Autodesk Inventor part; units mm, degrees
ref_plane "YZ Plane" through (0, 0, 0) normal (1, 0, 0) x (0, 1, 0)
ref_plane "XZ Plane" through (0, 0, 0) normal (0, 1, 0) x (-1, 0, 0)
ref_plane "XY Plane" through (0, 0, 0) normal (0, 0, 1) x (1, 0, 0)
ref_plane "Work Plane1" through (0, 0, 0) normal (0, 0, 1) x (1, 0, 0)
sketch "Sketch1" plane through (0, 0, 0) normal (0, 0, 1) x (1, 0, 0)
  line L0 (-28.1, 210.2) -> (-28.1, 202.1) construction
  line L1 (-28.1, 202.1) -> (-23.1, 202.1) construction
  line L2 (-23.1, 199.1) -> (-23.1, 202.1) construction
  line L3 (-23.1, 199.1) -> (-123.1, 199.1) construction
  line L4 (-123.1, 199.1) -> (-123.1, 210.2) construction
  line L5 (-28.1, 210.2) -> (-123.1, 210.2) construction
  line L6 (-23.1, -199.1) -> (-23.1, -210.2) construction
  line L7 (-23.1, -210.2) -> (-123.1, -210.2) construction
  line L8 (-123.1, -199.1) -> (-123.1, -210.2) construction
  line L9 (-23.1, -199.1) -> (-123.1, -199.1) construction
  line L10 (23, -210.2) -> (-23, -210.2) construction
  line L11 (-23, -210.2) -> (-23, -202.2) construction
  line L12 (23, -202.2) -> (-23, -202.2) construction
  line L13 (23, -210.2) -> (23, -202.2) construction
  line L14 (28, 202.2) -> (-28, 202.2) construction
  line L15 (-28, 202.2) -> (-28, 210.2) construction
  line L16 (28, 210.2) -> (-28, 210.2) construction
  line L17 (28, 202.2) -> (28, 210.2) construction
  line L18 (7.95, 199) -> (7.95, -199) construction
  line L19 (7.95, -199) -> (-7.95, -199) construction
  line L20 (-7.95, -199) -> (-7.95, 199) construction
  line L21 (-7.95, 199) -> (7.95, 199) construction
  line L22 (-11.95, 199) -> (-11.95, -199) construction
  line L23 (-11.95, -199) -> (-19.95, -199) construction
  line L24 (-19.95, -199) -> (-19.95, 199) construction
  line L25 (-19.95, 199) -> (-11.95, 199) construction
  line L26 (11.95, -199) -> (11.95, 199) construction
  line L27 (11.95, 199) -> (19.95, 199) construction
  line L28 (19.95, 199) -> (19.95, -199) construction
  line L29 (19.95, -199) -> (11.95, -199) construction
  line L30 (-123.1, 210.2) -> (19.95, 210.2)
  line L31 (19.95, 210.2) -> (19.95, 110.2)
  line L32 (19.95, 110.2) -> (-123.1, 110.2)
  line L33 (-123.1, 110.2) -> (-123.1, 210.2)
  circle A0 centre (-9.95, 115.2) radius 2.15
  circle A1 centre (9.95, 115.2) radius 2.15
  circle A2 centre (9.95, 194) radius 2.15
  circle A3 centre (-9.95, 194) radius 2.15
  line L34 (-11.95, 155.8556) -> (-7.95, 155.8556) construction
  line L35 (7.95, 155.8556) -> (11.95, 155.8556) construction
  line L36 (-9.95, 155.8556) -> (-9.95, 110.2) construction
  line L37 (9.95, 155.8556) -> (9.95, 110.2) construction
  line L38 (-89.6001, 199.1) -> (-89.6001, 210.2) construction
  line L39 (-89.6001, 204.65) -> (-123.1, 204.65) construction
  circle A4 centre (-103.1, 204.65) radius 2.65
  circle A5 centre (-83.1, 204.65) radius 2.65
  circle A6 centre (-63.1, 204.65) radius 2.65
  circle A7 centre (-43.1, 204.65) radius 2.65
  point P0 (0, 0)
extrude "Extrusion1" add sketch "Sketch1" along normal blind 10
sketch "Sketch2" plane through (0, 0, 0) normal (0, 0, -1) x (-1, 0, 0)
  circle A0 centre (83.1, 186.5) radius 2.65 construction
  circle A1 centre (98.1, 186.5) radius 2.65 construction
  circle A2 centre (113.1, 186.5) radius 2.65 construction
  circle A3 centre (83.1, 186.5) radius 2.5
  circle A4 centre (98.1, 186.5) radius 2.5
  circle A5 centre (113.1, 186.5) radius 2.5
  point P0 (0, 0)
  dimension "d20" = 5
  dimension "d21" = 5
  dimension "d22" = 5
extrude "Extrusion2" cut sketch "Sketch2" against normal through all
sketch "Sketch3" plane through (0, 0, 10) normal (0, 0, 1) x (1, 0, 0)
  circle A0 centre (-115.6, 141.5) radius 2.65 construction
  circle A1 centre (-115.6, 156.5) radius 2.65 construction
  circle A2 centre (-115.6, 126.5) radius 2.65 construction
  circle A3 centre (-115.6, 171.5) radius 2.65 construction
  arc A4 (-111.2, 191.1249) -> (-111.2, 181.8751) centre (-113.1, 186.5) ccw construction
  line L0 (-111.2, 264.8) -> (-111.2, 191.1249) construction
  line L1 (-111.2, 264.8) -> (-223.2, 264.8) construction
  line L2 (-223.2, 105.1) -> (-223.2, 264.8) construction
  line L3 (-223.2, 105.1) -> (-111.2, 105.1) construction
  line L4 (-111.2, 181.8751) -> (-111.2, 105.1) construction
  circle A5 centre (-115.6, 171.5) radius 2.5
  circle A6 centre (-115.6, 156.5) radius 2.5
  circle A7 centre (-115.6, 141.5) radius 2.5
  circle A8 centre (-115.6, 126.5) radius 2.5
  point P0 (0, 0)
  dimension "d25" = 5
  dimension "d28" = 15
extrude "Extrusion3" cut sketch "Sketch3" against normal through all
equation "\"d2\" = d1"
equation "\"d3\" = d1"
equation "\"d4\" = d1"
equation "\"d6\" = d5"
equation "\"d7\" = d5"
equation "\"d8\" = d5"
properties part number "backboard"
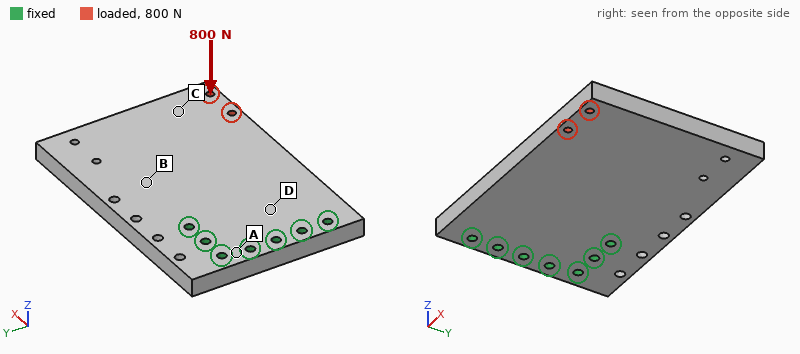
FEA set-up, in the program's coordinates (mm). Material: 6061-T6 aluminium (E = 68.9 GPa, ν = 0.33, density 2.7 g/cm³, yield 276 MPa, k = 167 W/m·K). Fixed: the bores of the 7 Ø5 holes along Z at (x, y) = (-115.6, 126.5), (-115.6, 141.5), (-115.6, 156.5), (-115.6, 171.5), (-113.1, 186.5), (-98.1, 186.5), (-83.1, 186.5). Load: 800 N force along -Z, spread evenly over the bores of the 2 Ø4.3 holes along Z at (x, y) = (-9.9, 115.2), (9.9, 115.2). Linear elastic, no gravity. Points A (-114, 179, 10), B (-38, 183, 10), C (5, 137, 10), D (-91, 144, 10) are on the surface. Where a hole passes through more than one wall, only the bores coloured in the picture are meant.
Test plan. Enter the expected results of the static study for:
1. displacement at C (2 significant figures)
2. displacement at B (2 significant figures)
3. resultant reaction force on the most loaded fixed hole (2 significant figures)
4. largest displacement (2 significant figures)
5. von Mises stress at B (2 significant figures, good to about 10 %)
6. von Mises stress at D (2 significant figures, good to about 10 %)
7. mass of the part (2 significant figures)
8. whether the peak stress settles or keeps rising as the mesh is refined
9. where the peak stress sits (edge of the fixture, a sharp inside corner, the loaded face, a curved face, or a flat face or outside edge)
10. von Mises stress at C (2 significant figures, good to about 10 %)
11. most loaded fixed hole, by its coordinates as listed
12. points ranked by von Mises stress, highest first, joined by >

0.58 mm
0.14 mm
1.6 kN
0.83 mm
25 MPa
36 MPa
380 g
keeps rising
edge of the fixture
15 MPa
(-83.1, 186.5)
D > B > C > A
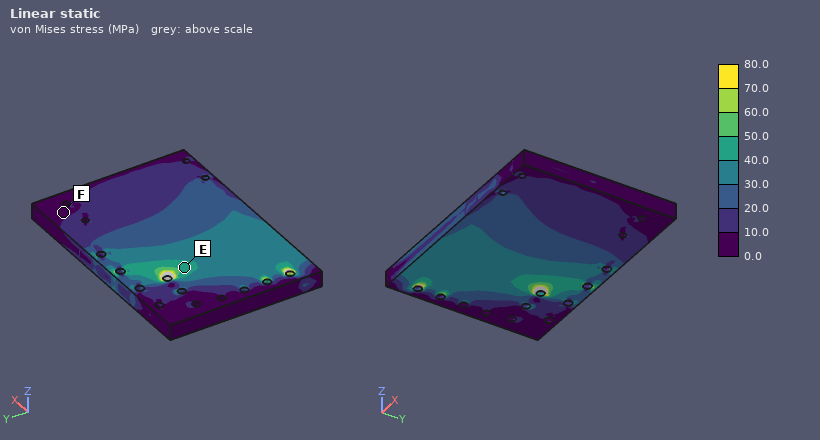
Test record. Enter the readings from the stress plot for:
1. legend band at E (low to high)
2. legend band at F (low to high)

40.0 to 50.0 MPa
0.0 to 10.0 MPa
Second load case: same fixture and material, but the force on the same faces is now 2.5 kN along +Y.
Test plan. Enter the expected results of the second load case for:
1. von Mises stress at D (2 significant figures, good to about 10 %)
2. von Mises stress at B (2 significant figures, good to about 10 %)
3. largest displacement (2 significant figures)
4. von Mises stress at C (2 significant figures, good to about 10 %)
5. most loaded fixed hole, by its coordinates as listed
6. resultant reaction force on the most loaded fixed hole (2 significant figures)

6.5 MPa
5.9 MPa
42 µm
5.6 MPa
(-83.1, 186.5)
3.4 kN
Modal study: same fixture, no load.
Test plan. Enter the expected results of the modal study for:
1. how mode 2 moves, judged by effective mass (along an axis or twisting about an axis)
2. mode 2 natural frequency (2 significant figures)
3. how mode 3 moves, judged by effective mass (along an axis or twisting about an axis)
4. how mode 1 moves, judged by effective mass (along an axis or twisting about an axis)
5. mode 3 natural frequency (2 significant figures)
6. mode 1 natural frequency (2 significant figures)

twisting about X
1500 Hz
along Z
along Z
3400 Hz
620 Hz
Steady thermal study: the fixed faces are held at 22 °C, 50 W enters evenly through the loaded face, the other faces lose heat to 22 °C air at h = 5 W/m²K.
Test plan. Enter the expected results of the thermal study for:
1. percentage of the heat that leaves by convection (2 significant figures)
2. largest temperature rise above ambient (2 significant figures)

4.9 %
49 K
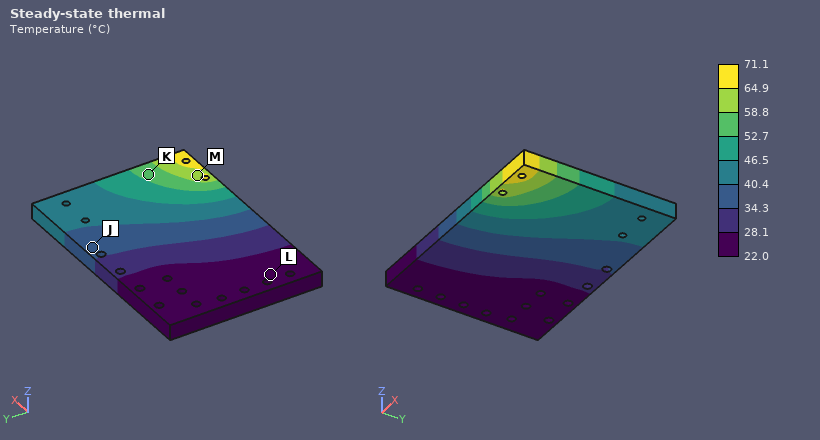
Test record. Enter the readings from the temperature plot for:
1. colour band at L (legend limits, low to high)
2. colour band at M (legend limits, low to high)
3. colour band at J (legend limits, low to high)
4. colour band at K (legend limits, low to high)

22.0 to 28.1 °C
58.8 to 64.9 °C
34.3 to 40.4 °C
52.7 to 58.8 °C
